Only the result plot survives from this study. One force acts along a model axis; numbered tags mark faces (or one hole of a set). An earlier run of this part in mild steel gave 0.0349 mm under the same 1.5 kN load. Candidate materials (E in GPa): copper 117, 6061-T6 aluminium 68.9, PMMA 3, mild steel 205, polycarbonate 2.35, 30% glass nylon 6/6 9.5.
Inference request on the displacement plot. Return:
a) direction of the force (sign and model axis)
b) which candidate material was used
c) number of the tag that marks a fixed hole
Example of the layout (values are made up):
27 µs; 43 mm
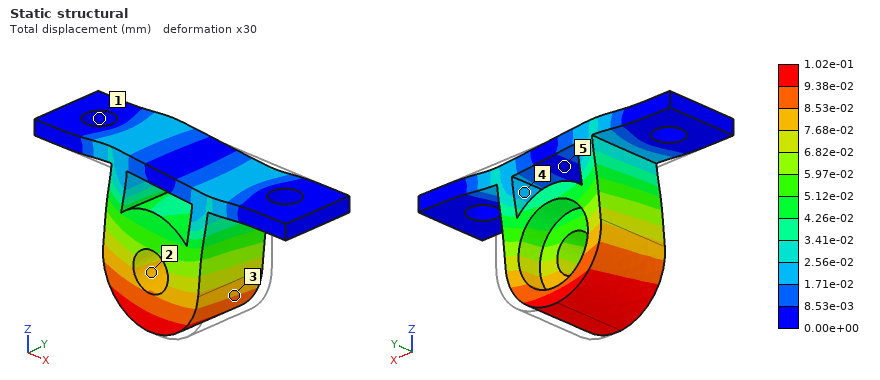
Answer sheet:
-X; 6061-T6 aluminium; 1
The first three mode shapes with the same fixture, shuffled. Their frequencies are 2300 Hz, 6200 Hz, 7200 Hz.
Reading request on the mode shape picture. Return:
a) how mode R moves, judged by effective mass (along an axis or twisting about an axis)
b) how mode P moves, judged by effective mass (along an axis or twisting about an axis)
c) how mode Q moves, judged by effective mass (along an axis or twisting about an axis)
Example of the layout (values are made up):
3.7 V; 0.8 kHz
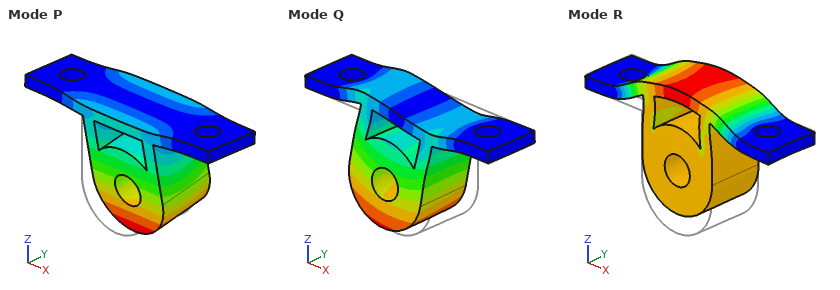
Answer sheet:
along Z; along Y; along X
